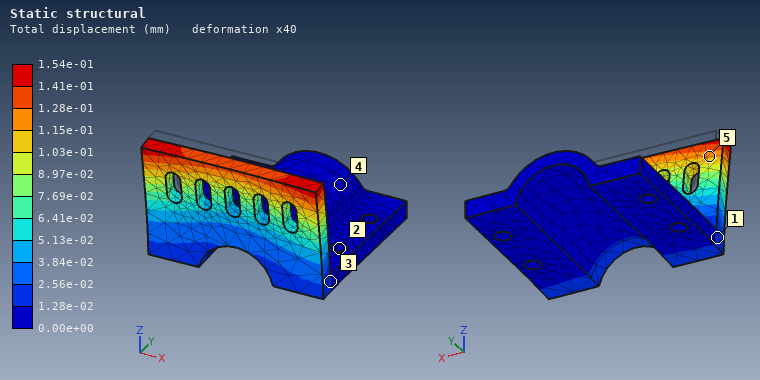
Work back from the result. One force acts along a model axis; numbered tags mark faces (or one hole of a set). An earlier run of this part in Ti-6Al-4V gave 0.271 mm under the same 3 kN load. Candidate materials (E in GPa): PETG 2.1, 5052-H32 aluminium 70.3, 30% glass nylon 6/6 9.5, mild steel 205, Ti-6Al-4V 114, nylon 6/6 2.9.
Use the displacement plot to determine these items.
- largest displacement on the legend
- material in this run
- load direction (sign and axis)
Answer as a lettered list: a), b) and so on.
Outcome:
a) 1.54e-01 mm
b) mild steel
c) -Y
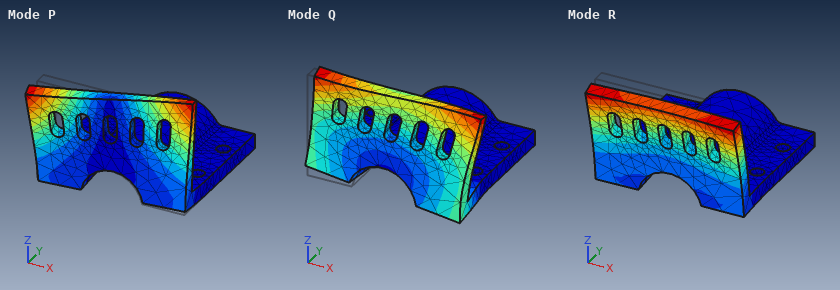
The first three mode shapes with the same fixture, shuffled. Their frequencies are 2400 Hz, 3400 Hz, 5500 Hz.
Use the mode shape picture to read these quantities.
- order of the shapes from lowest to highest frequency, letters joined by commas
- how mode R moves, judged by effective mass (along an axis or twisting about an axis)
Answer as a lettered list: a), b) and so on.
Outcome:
a) R, P, Q
b) along Y
